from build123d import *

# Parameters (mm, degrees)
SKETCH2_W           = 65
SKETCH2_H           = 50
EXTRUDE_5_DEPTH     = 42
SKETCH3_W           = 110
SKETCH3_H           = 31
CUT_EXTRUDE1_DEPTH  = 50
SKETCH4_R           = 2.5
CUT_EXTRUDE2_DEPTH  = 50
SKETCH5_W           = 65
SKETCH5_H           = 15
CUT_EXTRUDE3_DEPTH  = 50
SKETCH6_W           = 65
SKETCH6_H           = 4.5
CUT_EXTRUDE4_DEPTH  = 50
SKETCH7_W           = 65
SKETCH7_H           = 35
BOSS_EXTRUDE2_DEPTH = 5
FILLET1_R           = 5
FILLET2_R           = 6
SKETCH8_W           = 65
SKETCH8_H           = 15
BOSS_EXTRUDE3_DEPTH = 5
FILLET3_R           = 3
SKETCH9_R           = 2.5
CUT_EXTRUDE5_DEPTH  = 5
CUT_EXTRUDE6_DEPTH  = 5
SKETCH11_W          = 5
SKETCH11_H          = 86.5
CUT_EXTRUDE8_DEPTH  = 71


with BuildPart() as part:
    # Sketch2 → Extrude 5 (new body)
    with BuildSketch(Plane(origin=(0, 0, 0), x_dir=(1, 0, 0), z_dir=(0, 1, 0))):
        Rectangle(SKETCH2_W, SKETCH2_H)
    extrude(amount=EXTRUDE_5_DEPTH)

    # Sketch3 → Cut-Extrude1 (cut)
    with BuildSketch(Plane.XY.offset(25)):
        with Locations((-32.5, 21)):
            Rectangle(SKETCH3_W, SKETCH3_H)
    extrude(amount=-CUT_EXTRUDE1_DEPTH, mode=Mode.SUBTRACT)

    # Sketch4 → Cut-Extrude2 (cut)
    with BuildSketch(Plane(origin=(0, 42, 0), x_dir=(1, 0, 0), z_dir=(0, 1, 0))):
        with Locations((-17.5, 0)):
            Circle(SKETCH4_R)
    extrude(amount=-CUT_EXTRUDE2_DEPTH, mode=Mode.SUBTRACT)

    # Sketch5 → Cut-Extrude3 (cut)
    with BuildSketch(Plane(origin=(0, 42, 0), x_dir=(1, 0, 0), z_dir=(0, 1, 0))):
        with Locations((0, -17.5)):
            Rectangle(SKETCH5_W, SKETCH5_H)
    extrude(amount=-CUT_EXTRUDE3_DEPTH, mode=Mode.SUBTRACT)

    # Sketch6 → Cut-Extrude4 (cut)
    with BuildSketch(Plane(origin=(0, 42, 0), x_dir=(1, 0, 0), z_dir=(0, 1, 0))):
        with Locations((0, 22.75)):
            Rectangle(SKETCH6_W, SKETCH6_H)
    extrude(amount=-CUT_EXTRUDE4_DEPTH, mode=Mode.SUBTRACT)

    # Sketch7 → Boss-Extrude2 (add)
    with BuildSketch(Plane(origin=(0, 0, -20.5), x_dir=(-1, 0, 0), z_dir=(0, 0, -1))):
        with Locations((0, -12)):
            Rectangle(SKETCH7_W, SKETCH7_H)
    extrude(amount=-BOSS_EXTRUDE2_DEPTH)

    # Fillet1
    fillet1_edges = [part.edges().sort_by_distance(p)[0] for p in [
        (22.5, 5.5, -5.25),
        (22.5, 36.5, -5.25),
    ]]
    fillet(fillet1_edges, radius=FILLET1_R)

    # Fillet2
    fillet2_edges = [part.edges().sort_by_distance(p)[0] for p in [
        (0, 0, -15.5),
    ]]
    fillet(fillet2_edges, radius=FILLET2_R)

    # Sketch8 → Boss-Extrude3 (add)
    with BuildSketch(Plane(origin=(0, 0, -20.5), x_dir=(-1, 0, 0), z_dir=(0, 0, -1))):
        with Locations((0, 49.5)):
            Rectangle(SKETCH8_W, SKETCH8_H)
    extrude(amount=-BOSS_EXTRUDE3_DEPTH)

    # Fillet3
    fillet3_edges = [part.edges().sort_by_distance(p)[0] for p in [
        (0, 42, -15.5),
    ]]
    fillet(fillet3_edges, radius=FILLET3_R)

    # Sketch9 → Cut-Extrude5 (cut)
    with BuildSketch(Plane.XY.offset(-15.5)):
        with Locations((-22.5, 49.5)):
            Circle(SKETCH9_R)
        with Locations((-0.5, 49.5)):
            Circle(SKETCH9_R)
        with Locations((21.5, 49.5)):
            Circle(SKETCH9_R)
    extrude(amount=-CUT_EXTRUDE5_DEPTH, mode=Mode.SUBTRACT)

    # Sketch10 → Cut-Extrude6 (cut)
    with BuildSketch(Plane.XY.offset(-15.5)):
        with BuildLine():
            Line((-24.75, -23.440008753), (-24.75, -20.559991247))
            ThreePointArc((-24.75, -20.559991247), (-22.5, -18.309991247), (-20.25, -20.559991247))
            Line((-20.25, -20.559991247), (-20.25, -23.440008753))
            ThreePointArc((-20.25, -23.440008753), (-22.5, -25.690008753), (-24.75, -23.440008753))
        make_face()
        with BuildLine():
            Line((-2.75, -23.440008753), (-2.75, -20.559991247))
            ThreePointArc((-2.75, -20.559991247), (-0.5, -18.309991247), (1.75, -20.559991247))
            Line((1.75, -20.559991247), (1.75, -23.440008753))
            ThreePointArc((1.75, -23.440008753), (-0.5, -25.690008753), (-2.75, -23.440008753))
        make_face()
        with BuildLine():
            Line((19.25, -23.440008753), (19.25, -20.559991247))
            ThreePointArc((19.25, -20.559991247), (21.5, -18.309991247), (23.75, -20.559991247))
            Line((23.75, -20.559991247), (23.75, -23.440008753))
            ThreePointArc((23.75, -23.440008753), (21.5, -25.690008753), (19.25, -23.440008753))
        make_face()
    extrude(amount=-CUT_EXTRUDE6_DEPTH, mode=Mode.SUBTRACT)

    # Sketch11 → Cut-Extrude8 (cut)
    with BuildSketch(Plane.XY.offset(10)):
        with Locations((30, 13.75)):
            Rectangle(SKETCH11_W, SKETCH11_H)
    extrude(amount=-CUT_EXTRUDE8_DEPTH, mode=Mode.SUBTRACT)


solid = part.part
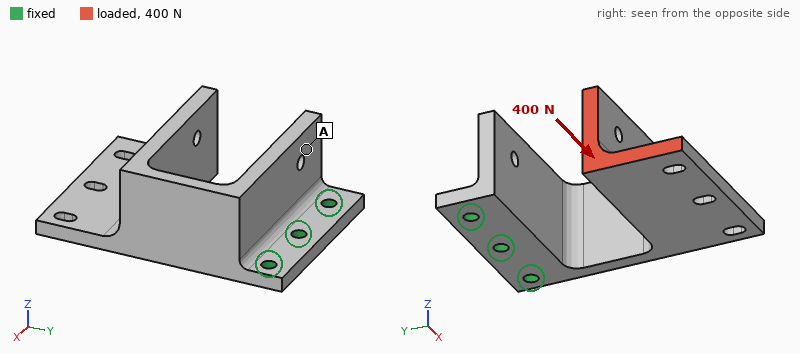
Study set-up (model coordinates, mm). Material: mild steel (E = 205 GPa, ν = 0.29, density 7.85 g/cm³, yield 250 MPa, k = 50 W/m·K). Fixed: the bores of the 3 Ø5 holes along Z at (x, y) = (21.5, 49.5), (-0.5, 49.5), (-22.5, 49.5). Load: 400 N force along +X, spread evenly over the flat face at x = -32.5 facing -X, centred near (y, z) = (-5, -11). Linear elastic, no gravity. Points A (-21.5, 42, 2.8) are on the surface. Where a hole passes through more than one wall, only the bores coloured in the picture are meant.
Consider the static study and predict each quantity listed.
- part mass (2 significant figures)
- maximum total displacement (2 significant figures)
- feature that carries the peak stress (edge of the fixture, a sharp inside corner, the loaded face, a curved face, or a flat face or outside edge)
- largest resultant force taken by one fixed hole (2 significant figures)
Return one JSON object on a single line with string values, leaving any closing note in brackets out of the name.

{"part mass": "300 g", "maximum total displacement": "0.47 mm", "feature that carries the peak stress": "a curved face", "largest resultant force taken by one fixed hole": "850 N"}
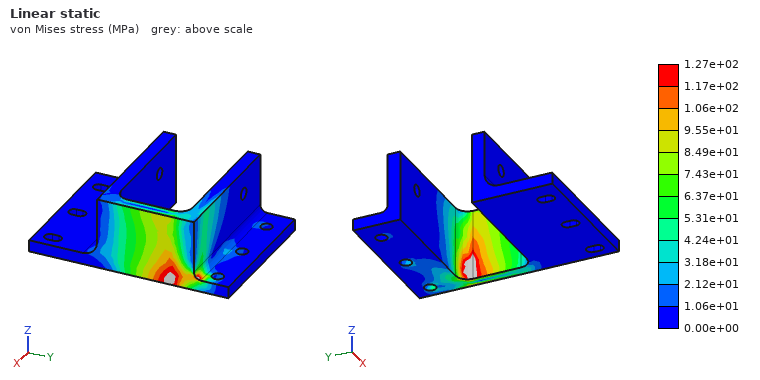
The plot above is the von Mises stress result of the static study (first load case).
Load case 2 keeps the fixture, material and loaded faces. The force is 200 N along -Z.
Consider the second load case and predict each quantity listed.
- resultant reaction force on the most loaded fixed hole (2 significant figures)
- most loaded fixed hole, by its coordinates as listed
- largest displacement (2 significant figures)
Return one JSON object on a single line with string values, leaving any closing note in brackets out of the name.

{"resultant reaction force on the most loaded fixed hole": "270 N", "most loaded fixed hole, by its coordinates as listed": "(-0.5, 49.5)", "largest displacement": "0.28 mm"}
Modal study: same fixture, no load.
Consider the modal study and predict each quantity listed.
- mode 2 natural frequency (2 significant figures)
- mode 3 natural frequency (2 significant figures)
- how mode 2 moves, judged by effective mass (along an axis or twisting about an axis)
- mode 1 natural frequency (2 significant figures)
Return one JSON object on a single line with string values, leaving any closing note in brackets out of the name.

{"mode 2 natural frequency": "520 Hz", "mode 3 natural frequency": "1400 Hz", "how mode 2 moves, judged by effective mass": "along Z", "mode 1 natural frequency": "410 Hz"}
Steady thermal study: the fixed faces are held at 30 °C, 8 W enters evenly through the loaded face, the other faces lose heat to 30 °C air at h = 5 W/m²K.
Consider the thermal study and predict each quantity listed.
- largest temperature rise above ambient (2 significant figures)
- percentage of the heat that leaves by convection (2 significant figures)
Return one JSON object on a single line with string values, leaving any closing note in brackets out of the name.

{"largest temperature rise above ambient": "66 K", "percentage of the heat that leaves by convection": "30 %"}
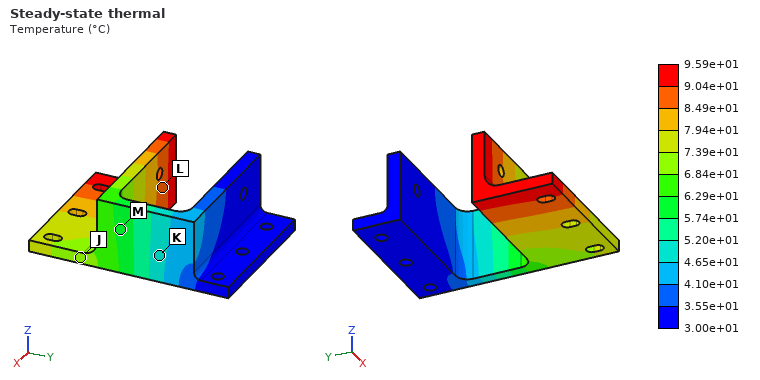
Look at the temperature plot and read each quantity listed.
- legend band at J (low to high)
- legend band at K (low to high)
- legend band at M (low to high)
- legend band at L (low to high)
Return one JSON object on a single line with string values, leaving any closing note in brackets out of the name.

{"legend band at J": "6.84e+01 to 7.39e+01 °C", "legend band at K": "4.65e+01 to 5.20e+01 °C", "legend band at M": "5.74e+01 to 6.29e+01 °C", "legend band at L": "8.49e+01 to 9.04e+01 °C"}
